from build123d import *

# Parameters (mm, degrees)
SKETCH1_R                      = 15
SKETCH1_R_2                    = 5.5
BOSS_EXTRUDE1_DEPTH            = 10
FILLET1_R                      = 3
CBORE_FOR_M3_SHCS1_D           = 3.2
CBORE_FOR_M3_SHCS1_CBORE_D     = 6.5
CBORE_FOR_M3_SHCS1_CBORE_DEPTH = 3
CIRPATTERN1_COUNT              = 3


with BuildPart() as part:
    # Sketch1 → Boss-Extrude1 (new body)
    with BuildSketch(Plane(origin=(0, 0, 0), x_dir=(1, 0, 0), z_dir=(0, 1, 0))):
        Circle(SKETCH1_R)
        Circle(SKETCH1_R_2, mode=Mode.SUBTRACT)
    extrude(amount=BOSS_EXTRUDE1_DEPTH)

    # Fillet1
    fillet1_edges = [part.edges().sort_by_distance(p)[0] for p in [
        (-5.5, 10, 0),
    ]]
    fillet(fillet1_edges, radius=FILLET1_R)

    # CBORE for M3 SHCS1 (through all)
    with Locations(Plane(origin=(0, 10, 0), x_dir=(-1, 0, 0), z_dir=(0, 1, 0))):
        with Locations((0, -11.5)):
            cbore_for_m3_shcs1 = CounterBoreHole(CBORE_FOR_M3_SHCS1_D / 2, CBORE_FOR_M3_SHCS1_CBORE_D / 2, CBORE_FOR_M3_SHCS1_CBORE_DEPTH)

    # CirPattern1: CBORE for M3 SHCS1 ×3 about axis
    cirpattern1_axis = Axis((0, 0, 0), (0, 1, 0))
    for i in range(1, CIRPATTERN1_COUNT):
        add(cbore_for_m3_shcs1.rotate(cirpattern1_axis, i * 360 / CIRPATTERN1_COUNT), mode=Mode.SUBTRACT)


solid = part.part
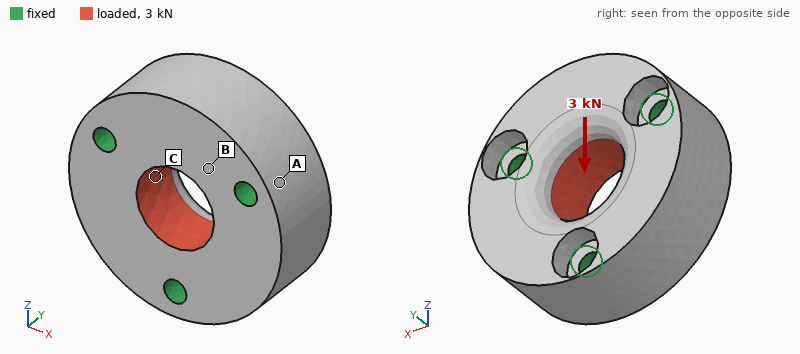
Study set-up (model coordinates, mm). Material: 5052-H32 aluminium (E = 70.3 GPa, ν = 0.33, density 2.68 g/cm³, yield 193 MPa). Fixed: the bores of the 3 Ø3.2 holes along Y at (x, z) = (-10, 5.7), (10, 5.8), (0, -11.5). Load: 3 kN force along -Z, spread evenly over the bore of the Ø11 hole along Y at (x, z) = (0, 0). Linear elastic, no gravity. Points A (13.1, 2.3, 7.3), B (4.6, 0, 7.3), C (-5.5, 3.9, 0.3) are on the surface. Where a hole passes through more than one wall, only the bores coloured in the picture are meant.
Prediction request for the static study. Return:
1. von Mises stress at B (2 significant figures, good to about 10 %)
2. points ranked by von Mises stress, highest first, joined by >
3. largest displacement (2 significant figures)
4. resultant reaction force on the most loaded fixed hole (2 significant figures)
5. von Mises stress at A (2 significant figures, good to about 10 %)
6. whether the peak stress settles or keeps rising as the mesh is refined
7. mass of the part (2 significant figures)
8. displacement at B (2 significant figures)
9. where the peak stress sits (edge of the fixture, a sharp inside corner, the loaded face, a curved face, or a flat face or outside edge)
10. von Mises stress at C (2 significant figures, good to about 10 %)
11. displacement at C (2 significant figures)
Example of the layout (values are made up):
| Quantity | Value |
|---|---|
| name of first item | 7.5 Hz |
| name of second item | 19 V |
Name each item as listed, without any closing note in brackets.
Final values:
| Quantity | Value |
|---|---|
| von Mises stress at B | 13 MPa |
| points ranked by von Mises stress, highest first, joined by > | C > B > A |
| largest displacement | 3.3 µm |
| resultant reaction force on the most loaded fixed hole | 1.1 kN |
| von Mises stress at A | 3.5 MPa |
| whether the peak stress settles or keeps rising as the mesh is refined | keeps rising |
| mass of the part | 15 g |
| displacement at B | 2.0 µm |
| where the peak stress sits | edge of the fixture |
| von Mises stress at C | 22 MPa |
| displacement at C | 2.1 µm |
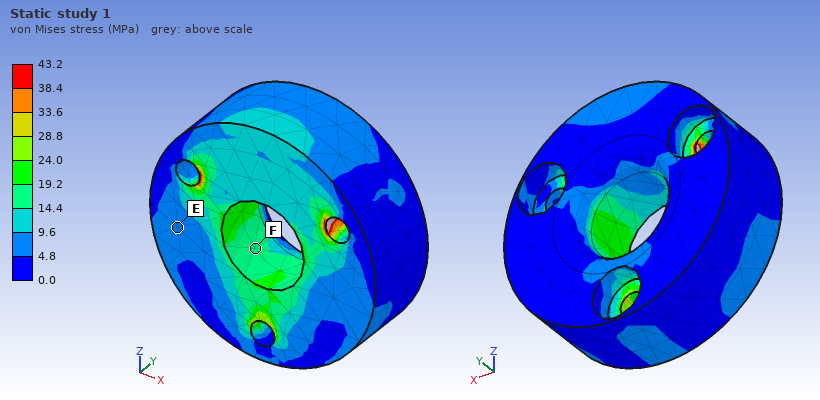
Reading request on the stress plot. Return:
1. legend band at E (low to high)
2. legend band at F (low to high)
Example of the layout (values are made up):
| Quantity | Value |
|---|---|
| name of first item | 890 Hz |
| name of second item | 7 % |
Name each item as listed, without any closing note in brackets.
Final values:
| Quantity | Value |
|---|---|
| legend band at E | 4.8 to 9.6 MPa |
| legend band at F | 14.4 to 19.2 MPa |
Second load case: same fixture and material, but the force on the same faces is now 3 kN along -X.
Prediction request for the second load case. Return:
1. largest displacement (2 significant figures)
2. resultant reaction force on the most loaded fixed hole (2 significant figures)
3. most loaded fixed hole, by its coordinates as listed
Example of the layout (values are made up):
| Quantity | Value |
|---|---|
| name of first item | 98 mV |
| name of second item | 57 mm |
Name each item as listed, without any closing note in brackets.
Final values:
| Quantity | Value |
|---|---|
| largest displacement | 3.0 µm |
| resultant reaction force on the most loaded fixed hole | 1.1 kN |
| most loaded fixed hole, by its coordinates as listed | (0, -11.5) |
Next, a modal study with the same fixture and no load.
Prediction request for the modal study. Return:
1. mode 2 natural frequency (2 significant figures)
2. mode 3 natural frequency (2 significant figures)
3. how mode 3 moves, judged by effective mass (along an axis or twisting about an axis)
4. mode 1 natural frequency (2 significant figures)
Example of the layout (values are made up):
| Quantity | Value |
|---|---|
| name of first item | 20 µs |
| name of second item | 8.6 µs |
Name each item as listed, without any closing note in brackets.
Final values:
| Quantity | Value |
|---|---|
| mode 2 natural frequency | 38 kHz |
| mode 3 natural frequency | 45 kHz |
| how mode 3 moves, judged by effective mass | along Y |
| mode 1 natural frequency | 38 kHz |
